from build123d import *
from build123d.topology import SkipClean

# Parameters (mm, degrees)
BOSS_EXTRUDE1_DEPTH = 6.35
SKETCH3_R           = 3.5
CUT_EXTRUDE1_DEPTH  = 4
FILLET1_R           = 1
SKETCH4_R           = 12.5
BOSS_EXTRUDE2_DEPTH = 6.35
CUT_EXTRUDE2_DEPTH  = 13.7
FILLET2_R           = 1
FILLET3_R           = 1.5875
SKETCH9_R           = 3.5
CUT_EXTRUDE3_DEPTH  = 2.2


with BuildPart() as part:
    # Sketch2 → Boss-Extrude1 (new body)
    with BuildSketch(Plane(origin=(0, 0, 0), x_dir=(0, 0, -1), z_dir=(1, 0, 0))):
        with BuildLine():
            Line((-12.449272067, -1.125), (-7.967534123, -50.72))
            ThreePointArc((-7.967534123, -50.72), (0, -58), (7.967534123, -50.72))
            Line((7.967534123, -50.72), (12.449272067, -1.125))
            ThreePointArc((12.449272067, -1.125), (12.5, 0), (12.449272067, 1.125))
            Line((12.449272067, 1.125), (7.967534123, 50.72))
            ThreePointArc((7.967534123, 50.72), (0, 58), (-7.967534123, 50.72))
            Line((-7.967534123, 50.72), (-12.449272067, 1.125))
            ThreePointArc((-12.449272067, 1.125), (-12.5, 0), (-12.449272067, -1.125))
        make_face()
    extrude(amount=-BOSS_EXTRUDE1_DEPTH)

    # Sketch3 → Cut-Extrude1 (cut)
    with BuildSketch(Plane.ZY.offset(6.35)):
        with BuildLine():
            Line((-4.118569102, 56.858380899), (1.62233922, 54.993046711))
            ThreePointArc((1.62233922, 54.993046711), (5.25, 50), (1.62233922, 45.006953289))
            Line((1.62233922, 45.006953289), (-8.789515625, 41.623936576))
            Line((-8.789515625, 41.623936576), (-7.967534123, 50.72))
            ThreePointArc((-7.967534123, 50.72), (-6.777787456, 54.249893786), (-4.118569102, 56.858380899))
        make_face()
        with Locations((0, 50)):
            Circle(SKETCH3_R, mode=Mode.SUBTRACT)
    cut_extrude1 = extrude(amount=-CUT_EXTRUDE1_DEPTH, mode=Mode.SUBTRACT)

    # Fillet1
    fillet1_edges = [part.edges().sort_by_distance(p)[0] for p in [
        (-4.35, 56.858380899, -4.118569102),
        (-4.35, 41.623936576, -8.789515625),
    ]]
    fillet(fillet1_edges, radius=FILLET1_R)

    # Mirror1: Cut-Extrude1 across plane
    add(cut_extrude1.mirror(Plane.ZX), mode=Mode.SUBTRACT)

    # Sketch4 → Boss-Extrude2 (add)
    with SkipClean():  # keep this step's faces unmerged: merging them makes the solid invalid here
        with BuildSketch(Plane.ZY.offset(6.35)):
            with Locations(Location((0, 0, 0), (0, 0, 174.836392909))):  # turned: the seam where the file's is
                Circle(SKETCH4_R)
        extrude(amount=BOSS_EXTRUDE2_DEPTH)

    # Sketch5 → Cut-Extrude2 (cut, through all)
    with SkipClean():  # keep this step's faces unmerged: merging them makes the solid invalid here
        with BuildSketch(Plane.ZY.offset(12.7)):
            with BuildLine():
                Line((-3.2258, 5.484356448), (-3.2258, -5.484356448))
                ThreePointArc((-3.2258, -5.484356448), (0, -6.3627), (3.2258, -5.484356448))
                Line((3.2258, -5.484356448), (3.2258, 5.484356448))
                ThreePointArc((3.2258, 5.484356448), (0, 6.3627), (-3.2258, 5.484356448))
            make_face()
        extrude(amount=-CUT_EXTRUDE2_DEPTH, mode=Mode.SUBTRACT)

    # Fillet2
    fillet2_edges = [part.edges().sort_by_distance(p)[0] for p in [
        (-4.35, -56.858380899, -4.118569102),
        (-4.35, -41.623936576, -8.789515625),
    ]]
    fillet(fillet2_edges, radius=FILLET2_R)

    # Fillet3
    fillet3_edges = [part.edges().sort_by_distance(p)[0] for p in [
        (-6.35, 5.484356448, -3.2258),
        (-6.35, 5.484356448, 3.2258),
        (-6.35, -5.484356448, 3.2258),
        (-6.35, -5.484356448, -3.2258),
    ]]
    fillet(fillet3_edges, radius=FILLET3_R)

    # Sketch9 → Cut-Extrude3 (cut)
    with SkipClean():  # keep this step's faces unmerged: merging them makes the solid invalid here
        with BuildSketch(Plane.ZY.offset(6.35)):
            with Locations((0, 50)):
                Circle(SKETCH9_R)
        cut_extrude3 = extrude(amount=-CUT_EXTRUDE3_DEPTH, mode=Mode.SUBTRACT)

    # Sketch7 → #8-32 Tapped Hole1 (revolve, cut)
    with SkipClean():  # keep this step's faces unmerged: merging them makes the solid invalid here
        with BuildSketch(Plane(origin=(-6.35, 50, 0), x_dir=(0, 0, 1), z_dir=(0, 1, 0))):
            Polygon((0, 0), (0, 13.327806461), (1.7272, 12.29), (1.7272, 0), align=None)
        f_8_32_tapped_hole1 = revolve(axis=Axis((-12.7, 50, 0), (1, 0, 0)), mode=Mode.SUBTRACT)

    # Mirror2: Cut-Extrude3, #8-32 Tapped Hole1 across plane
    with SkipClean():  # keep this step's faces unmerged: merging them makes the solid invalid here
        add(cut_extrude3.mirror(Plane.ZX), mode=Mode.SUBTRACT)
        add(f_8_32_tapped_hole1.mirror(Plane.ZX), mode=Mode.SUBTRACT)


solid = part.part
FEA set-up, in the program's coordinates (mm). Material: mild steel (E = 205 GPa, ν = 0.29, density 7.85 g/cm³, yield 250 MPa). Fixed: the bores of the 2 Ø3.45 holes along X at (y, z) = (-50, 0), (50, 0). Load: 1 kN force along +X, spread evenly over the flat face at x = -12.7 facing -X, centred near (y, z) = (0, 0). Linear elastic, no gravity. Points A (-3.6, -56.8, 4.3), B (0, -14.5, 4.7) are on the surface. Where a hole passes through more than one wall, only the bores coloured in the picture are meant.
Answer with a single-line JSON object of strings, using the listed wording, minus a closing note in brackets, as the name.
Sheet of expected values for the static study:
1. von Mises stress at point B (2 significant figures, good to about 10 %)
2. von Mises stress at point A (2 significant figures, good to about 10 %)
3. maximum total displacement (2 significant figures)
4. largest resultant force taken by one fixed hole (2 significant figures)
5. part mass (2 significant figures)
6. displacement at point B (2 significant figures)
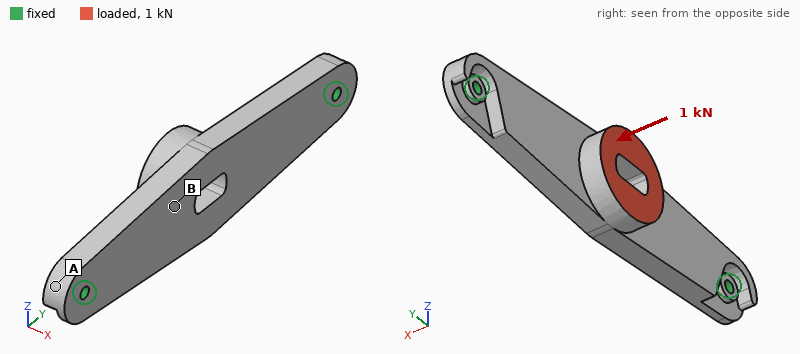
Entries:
{"von Mises stress at point B": "56 MPa", "von Mises stress at point A": "18 MPa", "maximum total displacement": "67 µm", "largest resultant force taken by one fixed hole": "1.5 kN", "part mass": "120 g", "displacement at point B": "61 µm"}
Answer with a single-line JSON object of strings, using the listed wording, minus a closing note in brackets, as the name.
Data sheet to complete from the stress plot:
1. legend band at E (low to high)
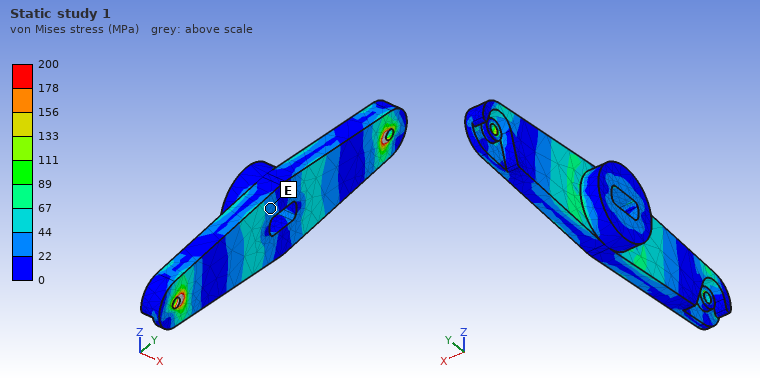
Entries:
{"legend band at E": "22 to 44 MPa"}
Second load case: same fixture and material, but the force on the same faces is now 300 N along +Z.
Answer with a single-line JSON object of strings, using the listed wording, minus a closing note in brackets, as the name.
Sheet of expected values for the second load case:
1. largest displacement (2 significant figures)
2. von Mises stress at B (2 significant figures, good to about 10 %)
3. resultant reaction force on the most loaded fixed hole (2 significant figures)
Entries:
{"largest displacement": "23 µm", "von Mises stress at B": "7.7 MPa", "resultant reaction force on the most loaded fixed hole": "150 N"}
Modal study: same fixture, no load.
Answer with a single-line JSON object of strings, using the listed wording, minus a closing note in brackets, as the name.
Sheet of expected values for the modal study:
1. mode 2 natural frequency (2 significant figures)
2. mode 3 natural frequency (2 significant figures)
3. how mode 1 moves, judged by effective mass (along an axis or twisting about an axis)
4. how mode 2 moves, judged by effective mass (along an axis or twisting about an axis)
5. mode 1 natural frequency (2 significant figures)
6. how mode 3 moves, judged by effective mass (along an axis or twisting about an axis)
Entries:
{"mode 2 natural frequency": "3300 Hz", "mode 3 natural frequency": "5500 Hz", "how mode 1 moves, judged by effective mass": "along X", "how mode 2 moves, judged by effective mass": "along Z", "mode 1 natural frequency": "2300 Hz", "how mode 3 moves, judged by effective mass": "along Z"}
